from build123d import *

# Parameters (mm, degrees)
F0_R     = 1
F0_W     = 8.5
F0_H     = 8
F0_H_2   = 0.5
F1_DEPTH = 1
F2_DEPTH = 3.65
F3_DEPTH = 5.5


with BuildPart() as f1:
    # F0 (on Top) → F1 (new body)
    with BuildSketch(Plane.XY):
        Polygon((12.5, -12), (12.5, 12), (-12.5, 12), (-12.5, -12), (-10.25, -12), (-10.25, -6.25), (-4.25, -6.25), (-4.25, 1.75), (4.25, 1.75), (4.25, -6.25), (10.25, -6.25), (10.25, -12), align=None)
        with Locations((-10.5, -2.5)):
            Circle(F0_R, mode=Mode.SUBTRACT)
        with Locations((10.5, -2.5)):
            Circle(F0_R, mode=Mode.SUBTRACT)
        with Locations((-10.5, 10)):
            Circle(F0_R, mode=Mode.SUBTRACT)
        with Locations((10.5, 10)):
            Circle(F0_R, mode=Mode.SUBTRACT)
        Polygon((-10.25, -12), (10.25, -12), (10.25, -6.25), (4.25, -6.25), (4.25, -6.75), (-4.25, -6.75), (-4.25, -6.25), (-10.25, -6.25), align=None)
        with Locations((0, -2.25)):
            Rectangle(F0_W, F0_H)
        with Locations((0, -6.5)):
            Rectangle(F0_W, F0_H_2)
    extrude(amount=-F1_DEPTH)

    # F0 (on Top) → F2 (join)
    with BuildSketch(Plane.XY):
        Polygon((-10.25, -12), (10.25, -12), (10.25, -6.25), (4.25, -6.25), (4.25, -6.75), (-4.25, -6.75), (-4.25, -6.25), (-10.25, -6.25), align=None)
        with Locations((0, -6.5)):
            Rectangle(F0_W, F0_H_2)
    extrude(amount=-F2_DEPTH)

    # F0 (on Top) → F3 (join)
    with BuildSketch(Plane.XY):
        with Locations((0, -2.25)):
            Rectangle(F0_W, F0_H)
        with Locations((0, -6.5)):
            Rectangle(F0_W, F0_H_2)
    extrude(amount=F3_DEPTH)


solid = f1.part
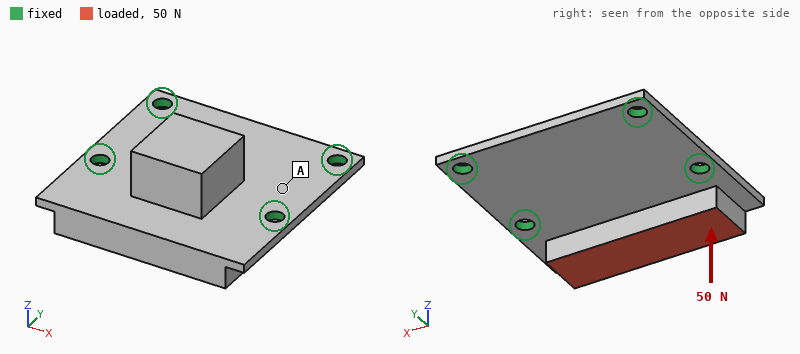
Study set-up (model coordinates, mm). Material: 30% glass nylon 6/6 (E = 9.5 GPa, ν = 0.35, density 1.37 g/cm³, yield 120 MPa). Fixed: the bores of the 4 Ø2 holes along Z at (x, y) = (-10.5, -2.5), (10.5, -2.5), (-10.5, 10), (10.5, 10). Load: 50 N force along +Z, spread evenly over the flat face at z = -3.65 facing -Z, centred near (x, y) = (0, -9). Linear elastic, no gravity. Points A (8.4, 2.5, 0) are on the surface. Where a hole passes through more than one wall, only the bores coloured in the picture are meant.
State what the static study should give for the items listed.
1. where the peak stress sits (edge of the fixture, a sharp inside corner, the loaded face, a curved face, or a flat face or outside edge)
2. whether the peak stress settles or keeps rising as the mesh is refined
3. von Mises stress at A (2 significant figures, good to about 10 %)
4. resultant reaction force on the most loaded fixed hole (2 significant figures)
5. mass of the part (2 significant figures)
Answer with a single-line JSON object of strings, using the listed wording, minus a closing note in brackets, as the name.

{"where the peak stress sits": "edge of the fixture", "whether the peak stress settles or keeps rising as the mesh is refined": "keeps rising", "von Mises stress at A": "7.2 MPa", "resultant reaction force on the most loaded fixed hole": "31 N", "mass of the part": "1.8 g"}
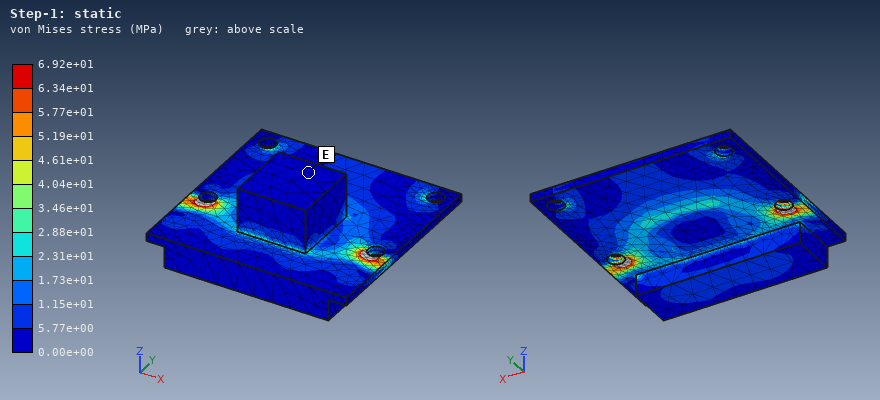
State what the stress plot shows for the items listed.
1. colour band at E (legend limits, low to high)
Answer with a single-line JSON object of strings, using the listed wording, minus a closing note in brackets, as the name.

{"colour band at E": "0.00e+00 to 5.77e+00 MPa"}
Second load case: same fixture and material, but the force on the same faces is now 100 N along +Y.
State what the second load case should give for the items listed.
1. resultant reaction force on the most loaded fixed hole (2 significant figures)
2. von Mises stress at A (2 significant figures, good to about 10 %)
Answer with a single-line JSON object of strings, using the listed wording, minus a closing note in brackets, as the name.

{"resultant reaction force on the most loaded fixed hole": "40 N", "von Mises stress at A": "8.2 MPa"}
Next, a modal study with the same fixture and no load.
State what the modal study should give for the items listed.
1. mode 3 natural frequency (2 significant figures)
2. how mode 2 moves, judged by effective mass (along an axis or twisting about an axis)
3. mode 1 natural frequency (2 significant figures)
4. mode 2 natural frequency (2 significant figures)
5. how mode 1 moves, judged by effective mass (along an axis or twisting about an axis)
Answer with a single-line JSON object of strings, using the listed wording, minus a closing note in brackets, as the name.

{"mode 3 natural frequency": "8800 Hz", "how mode 2 moves, judged by effective mass": "along Z", "mode 1 natural frequency": "3000 Hz", "mode 2 natural frequency": "5600 Hz", "how mode 1 moves, judged by effective mass": "along Z"}
